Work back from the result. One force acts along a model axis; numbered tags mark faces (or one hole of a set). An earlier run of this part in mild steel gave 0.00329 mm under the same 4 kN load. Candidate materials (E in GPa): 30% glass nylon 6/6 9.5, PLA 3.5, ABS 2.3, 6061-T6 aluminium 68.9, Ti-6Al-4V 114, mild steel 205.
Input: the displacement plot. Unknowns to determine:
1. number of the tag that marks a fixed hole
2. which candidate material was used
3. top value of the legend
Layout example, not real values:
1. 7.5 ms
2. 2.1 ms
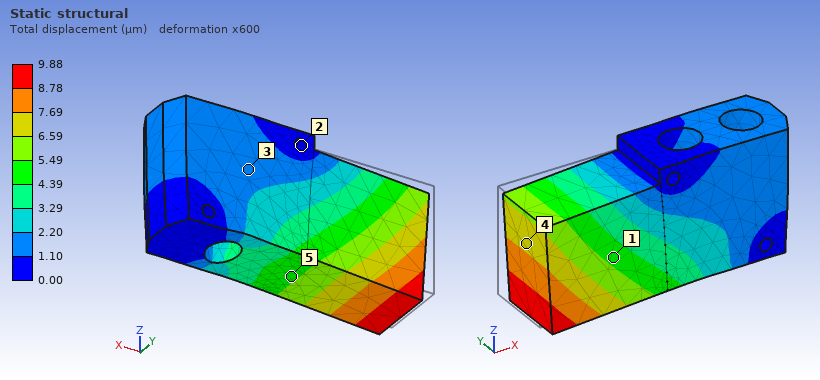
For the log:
1. 2
2. 6061-T6 aluminium
3. 9.88 µm
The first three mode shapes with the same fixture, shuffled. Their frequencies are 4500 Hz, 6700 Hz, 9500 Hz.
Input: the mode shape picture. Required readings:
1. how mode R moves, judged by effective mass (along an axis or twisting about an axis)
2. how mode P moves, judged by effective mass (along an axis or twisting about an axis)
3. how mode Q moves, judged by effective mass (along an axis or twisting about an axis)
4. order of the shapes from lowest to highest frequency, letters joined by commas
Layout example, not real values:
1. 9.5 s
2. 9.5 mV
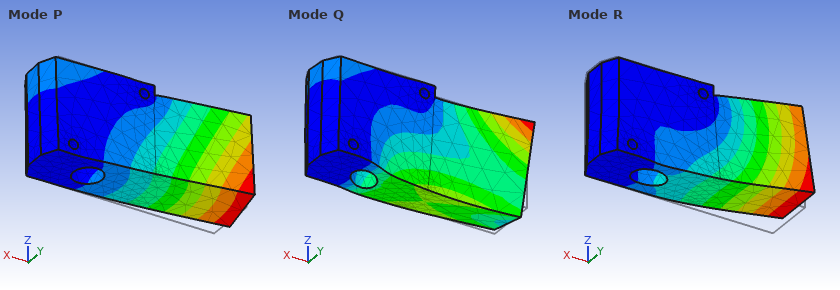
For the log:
1. along Z
2. along Y
3. twisting about X
4. P, R, Q
